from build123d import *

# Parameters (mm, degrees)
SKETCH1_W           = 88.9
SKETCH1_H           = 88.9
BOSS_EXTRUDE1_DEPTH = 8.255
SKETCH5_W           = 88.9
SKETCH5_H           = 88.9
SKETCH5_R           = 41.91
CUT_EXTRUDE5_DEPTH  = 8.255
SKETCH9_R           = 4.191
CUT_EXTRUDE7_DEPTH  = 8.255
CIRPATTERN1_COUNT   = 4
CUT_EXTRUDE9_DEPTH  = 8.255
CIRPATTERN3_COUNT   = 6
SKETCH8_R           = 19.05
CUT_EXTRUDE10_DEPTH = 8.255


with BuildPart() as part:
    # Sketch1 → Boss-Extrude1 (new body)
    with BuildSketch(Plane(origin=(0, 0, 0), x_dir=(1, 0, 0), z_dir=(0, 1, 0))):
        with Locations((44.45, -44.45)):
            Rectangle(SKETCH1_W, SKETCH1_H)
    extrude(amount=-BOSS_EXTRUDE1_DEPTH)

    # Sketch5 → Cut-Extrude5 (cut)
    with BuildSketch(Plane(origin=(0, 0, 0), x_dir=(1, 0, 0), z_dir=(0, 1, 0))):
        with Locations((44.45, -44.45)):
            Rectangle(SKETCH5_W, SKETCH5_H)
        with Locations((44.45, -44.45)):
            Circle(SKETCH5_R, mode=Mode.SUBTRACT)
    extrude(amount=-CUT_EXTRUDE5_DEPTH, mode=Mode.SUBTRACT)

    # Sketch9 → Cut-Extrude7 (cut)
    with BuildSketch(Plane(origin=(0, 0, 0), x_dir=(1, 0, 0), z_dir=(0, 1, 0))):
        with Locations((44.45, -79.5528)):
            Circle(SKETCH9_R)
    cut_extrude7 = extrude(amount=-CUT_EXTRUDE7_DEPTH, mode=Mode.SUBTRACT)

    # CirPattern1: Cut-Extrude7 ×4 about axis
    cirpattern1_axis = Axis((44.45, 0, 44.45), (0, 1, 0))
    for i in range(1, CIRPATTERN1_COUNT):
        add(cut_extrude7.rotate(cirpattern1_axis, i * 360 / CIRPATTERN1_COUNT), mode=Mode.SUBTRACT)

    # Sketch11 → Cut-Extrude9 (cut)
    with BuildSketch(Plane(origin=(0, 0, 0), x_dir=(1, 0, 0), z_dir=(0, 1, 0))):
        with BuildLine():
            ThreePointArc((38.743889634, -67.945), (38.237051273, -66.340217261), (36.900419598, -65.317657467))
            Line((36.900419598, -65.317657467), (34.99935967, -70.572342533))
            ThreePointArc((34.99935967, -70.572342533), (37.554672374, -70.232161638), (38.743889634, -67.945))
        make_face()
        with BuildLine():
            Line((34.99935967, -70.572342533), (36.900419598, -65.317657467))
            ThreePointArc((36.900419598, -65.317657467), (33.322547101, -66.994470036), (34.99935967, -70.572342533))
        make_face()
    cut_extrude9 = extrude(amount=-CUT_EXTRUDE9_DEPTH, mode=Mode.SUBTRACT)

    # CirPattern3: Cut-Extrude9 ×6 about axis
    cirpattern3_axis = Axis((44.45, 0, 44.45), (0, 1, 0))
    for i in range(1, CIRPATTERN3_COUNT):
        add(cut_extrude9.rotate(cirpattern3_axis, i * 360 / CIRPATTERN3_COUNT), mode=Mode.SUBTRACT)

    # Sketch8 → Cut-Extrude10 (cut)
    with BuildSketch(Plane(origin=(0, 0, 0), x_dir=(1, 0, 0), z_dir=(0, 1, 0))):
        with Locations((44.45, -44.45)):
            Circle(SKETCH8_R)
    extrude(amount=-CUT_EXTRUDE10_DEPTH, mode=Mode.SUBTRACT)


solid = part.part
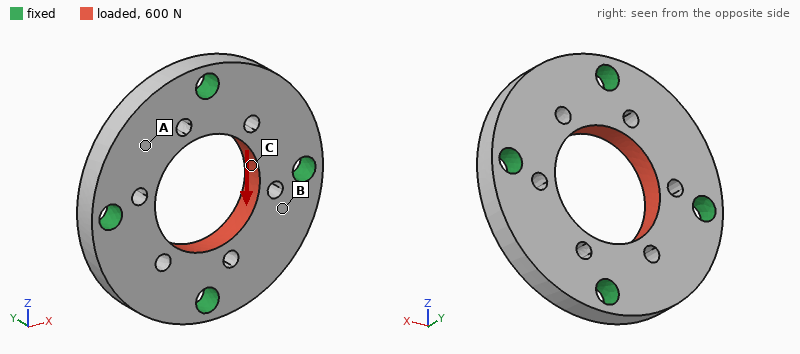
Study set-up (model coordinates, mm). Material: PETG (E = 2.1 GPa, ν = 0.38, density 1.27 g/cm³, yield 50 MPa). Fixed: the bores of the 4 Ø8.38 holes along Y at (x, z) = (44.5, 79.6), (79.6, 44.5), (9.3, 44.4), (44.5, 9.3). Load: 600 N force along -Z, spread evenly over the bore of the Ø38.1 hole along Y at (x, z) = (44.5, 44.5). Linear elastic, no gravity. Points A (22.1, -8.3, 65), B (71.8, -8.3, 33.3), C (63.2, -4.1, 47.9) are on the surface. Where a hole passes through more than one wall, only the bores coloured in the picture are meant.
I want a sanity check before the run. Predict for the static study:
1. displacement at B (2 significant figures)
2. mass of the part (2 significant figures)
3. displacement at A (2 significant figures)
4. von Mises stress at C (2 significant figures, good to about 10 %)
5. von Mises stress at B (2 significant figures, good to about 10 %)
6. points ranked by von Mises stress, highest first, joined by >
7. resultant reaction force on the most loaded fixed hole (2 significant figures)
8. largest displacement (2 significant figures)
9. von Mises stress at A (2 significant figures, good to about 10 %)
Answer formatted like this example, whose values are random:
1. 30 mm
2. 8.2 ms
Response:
1. 6.6 µm
2. 42 g
3. 10 µm
4. 1.0 MPa
5. 0.63 MPa
6. C > B > A
7. 160 N
8. 15 µm
9. 0.31 MPa
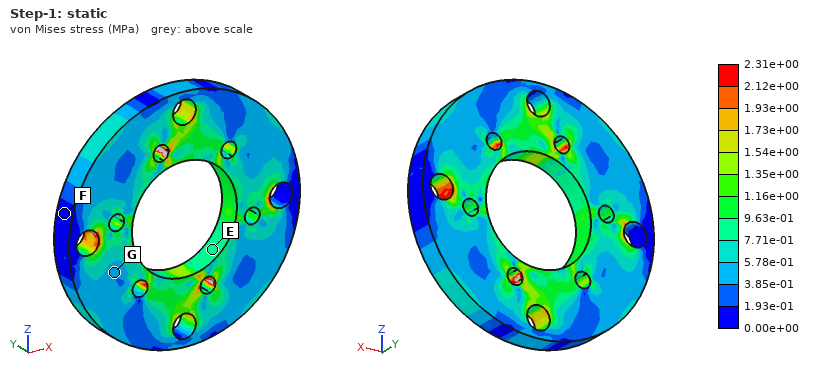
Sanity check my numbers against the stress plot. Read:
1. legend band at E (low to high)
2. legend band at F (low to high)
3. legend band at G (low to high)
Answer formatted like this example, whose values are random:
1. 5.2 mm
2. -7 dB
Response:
1. 7.71e-01 to 9.63e-01 MPa
2. 0.00e+00 to 1.93e-01 MPa
3. 3.85e-01 to 5.78e-01 MPa
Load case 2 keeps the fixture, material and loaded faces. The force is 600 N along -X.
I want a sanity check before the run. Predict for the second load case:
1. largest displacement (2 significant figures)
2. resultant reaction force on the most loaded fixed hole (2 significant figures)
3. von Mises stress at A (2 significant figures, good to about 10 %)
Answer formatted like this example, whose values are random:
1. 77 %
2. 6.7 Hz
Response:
1. 15 µm
2. 160 N
3. 0.31 MPa
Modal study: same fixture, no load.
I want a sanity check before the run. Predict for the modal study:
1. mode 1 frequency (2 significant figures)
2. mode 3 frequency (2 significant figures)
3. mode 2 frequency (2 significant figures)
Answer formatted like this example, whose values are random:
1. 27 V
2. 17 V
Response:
1. 3500 Hz
2. 3700 Hz
3. 3600 Hz
